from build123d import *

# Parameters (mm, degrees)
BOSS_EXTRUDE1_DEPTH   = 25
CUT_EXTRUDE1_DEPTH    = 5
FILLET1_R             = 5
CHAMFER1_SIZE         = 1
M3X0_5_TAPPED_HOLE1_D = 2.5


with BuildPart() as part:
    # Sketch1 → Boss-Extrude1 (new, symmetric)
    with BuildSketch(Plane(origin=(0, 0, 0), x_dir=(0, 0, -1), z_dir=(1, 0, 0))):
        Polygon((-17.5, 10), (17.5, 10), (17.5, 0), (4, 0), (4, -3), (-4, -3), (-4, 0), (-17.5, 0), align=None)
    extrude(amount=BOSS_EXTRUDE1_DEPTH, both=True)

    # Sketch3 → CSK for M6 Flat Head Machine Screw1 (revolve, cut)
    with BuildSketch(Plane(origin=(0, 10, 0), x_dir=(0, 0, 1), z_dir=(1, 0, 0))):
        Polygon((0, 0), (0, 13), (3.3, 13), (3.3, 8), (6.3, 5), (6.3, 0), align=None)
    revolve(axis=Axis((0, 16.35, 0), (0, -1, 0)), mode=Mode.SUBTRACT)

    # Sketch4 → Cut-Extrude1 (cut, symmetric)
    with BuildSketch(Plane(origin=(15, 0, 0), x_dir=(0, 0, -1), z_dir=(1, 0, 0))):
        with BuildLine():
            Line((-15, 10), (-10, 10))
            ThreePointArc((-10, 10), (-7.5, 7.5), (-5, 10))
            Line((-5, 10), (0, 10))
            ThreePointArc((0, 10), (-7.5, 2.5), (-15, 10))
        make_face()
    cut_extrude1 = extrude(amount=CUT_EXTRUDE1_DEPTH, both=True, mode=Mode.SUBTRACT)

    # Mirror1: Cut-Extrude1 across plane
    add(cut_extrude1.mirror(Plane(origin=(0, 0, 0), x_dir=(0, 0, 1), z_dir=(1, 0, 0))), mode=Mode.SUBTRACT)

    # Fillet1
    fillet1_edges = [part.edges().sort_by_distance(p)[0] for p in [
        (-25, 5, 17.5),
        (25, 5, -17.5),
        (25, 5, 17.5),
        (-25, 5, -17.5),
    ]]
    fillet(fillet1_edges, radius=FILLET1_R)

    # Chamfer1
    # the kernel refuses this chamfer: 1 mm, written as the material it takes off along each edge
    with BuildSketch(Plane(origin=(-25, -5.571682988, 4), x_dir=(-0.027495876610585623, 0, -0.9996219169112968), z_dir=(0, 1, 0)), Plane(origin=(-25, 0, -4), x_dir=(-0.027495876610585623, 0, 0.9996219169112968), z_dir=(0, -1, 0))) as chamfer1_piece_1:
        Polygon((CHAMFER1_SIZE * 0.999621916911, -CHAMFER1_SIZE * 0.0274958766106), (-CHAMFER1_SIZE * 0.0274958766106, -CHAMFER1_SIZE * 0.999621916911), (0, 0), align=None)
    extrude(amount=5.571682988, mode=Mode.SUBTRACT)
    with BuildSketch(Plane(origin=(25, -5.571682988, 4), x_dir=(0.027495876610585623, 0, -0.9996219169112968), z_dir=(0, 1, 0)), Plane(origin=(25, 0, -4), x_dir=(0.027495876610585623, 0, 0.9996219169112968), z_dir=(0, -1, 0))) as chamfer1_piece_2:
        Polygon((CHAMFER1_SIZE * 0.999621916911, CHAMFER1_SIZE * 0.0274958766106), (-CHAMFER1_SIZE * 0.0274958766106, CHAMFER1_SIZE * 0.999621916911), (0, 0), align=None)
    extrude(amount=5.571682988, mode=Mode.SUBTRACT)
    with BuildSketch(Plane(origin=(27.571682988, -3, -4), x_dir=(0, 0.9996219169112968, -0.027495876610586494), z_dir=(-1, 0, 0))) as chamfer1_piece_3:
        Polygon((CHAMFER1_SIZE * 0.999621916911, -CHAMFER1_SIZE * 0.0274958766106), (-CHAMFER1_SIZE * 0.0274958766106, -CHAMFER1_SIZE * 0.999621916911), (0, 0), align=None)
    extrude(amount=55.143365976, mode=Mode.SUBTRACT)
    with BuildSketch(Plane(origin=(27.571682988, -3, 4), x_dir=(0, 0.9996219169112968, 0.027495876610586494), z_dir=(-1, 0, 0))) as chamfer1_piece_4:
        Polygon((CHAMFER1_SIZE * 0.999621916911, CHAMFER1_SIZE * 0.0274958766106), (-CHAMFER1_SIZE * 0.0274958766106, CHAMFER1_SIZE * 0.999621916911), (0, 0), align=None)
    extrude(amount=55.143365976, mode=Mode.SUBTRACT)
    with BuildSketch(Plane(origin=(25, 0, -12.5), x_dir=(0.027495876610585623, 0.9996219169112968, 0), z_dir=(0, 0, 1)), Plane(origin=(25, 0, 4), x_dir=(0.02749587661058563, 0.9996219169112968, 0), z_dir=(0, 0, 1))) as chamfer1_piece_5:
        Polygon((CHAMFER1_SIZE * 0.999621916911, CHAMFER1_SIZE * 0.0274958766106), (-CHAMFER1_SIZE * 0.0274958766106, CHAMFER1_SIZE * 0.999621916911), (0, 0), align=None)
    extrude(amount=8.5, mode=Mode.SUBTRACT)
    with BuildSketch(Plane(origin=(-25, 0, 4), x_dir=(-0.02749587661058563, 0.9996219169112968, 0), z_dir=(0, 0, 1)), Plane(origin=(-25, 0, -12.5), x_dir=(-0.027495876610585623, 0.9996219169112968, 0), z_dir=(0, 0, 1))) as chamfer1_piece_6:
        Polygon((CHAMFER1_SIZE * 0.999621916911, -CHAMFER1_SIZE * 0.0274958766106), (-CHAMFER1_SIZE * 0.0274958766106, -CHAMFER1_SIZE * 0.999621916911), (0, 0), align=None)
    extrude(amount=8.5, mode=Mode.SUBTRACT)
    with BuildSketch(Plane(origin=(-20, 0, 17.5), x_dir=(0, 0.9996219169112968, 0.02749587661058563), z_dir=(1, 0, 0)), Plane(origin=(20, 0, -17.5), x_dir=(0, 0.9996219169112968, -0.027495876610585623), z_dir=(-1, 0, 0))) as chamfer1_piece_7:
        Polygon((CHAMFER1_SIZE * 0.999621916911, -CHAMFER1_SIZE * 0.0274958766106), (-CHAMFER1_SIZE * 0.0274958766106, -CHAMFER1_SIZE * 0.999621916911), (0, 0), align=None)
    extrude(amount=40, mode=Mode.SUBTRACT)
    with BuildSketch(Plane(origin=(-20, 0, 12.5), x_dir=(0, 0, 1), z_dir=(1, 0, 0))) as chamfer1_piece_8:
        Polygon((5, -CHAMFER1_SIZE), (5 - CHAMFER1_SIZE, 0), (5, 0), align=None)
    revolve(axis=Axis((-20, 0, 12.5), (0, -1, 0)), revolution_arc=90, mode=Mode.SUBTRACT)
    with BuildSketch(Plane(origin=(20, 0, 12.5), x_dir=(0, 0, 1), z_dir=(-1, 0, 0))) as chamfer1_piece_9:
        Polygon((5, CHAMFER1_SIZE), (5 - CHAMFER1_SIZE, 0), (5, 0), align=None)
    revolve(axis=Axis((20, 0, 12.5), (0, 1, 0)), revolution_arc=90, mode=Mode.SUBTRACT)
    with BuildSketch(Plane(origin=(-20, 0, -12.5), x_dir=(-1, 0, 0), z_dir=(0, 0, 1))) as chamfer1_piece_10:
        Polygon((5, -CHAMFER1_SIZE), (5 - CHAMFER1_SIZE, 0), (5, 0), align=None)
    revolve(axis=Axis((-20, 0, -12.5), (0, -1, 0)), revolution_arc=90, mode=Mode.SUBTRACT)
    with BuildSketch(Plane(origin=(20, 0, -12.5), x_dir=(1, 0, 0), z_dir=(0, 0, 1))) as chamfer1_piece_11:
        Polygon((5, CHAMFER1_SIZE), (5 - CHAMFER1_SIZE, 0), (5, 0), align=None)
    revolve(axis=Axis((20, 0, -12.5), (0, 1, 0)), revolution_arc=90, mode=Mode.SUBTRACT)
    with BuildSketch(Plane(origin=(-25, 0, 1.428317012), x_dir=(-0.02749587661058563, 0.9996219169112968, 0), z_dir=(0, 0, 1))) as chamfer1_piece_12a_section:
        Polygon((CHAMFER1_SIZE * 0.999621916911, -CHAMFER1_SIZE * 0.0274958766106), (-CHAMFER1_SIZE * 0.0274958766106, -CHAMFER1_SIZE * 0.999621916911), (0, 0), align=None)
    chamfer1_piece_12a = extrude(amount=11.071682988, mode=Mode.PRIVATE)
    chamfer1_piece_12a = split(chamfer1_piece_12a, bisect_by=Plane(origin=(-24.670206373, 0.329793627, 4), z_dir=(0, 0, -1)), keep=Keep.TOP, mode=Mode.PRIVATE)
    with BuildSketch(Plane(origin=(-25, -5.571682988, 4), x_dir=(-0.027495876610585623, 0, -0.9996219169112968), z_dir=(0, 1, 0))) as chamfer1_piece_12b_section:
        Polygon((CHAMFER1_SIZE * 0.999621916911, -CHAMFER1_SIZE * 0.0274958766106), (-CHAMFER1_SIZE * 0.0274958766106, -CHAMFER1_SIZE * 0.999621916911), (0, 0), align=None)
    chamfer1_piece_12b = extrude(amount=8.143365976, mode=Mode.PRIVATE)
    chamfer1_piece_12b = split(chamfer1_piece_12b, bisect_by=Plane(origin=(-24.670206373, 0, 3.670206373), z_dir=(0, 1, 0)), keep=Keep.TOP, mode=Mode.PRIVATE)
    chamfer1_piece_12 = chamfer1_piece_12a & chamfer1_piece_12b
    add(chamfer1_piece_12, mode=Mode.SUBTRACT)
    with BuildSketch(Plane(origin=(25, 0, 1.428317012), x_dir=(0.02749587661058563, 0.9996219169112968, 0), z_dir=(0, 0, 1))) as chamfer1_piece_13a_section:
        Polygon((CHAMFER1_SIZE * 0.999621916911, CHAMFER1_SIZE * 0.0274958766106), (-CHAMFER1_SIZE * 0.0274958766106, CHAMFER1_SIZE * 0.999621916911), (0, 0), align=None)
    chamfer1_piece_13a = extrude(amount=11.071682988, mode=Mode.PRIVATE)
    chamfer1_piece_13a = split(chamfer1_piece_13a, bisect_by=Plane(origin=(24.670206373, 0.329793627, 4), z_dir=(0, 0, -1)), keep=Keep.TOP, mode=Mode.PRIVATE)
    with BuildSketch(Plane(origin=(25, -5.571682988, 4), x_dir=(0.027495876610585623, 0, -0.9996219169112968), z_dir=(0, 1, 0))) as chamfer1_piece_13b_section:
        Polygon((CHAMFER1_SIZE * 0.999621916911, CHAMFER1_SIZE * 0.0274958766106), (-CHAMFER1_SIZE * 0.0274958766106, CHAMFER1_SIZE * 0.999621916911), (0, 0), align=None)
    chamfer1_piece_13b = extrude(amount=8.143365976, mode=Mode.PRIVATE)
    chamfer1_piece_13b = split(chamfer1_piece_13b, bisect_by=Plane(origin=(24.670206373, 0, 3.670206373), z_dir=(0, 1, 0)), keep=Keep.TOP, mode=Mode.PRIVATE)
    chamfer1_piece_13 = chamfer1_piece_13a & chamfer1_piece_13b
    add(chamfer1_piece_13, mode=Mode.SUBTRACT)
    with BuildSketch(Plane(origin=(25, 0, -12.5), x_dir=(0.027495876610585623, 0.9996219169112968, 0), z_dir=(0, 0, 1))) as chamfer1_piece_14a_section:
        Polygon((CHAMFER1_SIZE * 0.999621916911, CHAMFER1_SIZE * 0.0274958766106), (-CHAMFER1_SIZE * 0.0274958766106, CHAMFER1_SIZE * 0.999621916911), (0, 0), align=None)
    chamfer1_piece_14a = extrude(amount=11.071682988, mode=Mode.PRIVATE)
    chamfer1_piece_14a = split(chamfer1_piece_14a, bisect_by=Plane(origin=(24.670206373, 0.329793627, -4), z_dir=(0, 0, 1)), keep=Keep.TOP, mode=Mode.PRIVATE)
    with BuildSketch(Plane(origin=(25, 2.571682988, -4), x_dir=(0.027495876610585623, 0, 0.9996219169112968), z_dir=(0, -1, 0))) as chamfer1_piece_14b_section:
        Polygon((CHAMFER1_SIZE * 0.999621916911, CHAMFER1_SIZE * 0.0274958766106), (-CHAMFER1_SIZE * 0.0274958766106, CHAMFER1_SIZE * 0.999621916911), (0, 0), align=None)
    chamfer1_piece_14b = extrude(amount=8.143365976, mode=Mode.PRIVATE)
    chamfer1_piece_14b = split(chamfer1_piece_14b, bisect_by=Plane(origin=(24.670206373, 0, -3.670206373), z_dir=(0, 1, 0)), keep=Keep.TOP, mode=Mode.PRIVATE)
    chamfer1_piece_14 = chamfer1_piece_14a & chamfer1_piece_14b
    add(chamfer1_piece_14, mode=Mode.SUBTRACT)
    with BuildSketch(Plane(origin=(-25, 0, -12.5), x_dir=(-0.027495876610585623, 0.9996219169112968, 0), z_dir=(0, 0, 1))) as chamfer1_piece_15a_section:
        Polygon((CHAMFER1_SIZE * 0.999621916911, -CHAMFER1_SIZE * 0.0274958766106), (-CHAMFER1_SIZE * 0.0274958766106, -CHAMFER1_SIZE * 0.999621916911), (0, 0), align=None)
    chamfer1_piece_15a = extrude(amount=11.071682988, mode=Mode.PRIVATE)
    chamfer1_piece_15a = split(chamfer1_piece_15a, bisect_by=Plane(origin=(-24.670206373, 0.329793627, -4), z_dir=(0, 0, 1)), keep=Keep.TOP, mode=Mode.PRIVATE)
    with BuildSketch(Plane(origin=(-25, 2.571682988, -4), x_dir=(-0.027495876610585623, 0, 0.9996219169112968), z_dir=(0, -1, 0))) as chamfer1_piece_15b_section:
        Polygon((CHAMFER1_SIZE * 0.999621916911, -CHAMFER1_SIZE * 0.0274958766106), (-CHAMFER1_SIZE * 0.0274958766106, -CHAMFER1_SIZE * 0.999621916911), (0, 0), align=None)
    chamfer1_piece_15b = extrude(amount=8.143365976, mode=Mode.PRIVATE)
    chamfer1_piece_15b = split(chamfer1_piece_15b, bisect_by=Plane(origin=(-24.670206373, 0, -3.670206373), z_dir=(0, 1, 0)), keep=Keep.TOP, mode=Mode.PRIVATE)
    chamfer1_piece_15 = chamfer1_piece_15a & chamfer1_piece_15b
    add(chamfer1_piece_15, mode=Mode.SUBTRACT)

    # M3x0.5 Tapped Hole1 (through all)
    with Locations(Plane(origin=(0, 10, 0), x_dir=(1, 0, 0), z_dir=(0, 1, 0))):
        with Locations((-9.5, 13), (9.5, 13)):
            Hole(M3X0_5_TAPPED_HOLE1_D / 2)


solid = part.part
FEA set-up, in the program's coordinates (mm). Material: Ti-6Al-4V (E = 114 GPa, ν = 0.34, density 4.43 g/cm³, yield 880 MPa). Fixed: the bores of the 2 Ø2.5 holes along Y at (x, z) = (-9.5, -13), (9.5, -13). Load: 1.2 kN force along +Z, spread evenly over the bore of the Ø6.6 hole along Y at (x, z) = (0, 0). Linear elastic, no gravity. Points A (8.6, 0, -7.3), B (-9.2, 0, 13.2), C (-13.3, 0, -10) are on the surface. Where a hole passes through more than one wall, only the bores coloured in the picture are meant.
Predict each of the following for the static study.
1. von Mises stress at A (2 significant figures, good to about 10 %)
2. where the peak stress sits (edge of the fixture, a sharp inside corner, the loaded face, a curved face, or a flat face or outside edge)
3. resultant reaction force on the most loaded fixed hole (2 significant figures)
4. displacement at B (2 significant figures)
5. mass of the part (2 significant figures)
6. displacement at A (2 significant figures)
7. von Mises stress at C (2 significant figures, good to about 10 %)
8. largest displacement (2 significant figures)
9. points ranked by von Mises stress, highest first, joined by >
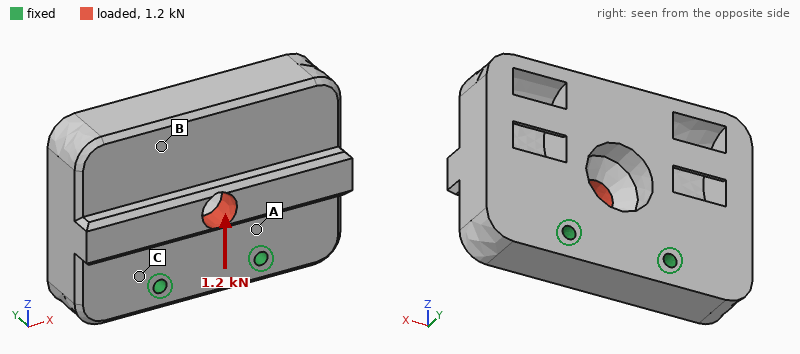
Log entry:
18 MPa
a flat face or outside edge
620 N
6.6 µm
69 g
1.4 µm
9.8 MPa
8.8 µm
A > C > B
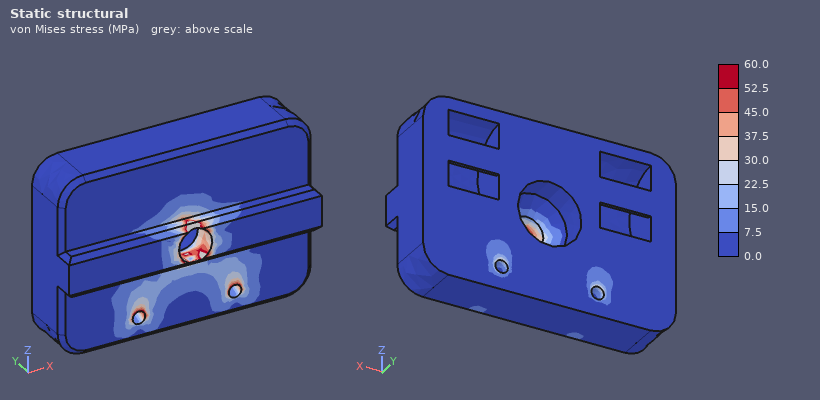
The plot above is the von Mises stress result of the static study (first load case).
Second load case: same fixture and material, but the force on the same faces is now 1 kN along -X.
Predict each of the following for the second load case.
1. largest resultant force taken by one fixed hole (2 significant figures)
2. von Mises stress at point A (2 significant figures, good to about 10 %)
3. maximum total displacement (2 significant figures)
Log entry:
810 N
11 MPa
4.8 µm
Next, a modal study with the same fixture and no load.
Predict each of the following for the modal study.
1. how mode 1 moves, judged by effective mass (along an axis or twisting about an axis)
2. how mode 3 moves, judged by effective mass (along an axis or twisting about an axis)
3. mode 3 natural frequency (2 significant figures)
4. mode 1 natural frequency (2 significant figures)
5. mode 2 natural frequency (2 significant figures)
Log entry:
along Y
along X
10 kHz
6300 Hz
9200 Hz
